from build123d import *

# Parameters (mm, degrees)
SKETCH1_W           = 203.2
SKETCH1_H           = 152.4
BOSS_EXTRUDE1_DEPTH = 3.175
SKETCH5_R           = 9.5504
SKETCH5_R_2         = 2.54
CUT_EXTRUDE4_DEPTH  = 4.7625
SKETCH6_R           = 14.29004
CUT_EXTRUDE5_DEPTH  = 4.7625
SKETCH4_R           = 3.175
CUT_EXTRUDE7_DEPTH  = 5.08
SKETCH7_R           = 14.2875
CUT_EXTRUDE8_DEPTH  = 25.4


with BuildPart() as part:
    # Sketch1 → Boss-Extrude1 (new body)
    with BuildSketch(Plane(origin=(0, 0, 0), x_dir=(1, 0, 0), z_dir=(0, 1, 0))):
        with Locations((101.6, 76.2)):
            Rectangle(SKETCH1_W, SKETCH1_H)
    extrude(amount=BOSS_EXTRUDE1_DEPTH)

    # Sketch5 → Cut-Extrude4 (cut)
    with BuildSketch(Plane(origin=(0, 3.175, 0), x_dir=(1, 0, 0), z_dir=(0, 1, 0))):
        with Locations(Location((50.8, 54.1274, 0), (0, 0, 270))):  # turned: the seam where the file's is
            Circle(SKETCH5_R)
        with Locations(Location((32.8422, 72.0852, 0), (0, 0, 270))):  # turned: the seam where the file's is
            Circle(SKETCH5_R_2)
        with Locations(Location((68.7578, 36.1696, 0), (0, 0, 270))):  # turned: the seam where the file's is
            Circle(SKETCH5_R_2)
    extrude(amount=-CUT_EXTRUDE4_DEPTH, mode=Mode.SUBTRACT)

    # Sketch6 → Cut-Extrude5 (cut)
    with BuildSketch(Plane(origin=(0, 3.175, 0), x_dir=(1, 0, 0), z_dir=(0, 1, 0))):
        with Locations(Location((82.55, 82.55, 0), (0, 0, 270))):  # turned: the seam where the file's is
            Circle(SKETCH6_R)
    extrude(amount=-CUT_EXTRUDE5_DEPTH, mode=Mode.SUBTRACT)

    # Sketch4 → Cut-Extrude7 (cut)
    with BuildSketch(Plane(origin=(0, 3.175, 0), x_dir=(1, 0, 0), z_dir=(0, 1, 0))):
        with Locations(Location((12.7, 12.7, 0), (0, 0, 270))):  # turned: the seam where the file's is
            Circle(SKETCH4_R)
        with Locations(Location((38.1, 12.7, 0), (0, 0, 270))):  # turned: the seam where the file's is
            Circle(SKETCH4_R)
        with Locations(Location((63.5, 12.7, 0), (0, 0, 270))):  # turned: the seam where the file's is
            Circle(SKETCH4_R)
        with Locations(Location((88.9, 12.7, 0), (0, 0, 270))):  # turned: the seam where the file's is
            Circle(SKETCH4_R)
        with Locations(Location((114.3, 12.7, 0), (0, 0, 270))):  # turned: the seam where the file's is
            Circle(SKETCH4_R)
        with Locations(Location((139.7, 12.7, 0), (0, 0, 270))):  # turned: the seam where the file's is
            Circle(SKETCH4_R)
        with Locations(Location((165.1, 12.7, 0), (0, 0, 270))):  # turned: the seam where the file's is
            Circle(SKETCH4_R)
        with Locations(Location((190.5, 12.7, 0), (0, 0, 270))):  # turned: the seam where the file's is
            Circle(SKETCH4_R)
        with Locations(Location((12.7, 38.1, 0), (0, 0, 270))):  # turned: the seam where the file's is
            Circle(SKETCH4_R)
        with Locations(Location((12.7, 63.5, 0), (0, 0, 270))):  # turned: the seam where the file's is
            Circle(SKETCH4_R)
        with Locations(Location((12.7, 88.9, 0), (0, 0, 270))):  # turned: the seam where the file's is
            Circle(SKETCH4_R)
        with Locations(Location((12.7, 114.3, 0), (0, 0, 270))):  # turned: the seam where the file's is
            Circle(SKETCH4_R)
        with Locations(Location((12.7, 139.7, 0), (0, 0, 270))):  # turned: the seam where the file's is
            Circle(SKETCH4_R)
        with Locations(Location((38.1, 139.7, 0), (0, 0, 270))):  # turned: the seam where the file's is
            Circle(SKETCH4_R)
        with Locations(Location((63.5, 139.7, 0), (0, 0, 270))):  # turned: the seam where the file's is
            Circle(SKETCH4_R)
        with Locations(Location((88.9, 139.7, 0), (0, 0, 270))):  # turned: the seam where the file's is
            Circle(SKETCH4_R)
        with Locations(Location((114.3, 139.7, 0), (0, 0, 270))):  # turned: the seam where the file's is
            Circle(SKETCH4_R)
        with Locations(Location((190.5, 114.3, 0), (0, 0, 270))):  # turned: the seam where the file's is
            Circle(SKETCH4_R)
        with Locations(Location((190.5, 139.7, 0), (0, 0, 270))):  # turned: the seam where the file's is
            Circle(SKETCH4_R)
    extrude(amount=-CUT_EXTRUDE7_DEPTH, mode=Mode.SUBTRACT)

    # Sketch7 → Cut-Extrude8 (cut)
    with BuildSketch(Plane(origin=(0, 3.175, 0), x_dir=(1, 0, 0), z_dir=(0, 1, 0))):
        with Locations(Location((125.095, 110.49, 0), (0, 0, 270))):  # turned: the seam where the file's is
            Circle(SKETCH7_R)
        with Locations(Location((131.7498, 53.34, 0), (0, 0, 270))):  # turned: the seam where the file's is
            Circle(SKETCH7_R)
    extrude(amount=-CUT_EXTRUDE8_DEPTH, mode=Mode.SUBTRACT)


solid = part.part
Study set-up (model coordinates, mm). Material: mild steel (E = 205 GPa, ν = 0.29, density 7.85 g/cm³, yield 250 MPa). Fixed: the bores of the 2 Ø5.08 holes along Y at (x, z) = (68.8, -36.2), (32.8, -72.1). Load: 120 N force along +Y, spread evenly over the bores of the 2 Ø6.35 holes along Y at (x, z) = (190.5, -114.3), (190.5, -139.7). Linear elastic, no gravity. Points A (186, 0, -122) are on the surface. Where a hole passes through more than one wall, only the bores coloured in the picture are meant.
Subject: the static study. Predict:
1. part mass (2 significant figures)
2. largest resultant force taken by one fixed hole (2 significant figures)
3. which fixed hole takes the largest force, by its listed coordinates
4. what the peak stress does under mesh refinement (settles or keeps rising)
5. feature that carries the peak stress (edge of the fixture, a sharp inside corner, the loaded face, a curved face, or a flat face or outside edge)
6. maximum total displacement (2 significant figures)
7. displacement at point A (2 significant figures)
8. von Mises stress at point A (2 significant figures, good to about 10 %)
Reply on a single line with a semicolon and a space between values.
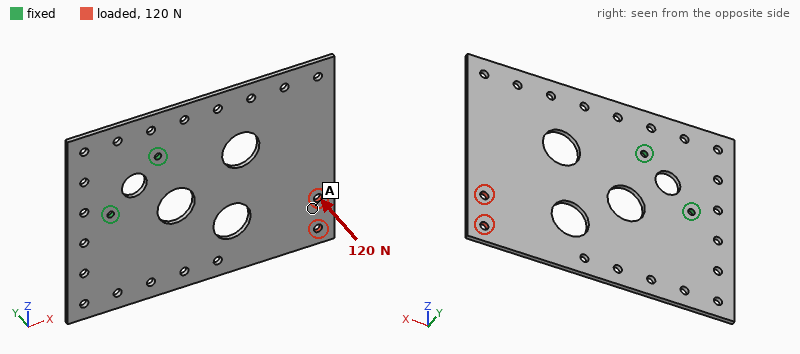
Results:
700 g; 130 N; (68.8, -36.2); keeps rising; edge of the fixture; 3.0 mm; 2.3 mm; 17 MPa
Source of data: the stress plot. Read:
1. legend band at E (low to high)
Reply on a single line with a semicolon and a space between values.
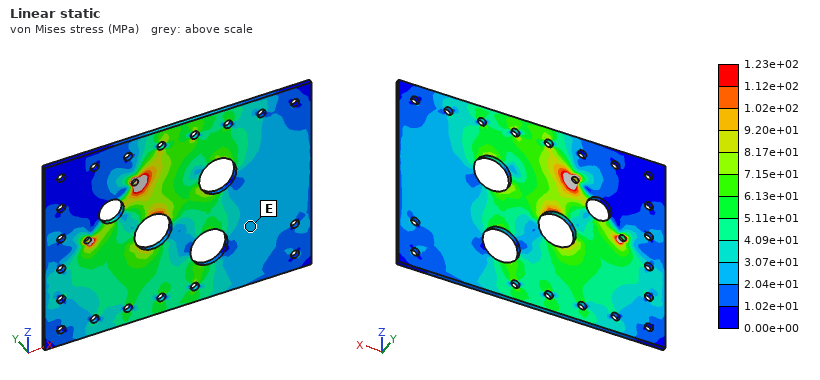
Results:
2.04e+01 to 3.07e+01 MPa
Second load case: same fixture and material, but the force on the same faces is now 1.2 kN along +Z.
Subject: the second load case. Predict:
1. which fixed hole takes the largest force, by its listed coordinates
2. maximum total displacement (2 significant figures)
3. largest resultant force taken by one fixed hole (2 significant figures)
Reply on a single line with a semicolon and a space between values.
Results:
(68.8, -36.2); 56 µm; 3.6 kN
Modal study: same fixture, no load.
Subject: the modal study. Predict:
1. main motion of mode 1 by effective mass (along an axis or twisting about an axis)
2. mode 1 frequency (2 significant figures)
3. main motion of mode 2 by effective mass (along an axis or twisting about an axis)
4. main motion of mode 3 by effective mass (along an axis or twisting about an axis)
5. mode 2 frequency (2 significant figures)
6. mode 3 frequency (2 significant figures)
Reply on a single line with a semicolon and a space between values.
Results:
along Y; 100 Hz; twisting about X; along Y; 220 Hz; 410 Hz
